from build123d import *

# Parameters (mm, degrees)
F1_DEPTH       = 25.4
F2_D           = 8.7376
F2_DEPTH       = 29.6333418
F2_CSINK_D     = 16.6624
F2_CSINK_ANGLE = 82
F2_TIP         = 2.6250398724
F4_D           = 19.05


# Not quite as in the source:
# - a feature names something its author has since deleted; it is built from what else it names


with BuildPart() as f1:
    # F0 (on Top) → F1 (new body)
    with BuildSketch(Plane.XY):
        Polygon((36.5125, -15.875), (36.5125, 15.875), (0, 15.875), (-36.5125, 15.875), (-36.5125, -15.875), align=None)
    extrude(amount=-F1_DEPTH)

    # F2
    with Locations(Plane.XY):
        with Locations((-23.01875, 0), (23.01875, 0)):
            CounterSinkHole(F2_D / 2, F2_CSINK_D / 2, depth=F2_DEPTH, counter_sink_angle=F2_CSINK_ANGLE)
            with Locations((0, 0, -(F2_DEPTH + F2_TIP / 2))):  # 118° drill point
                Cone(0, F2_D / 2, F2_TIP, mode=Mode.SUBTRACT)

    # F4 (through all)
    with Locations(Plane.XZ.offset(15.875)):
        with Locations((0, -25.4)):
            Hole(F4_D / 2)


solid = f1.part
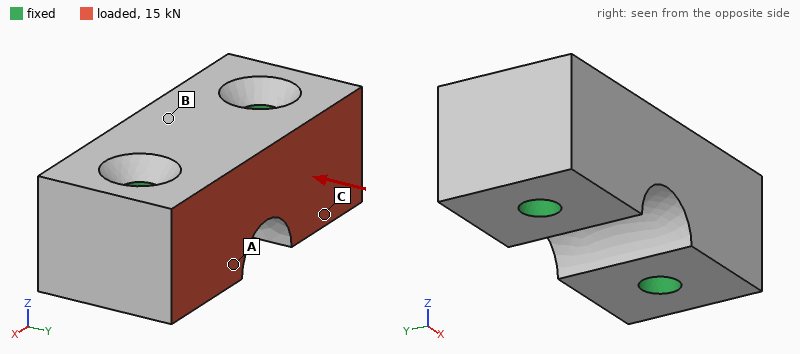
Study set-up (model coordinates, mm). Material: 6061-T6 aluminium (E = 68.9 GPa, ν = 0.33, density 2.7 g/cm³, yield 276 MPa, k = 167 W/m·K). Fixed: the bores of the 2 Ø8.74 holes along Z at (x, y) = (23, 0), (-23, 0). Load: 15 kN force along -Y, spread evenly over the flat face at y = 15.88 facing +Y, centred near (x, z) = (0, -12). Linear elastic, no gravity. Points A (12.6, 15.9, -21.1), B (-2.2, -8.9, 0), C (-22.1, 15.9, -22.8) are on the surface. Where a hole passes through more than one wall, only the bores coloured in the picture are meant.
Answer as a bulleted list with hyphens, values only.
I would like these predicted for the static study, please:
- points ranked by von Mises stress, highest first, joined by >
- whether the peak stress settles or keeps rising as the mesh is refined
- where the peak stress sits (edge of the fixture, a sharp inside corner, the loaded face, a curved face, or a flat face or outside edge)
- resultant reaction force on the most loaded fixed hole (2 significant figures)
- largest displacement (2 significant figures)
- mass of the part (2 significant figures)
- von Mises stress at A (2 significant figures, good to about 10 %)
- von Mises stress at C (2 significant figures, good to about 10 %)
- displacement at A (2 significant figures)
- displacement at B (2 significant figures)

- C > A > B
- keeps rising
- edge of the fixture
- 7.5 kN
- 6.9 µm
- 140 g
- 8.9 MPa
- 13 MPa
- 3.4 µm
- 4.4 µm
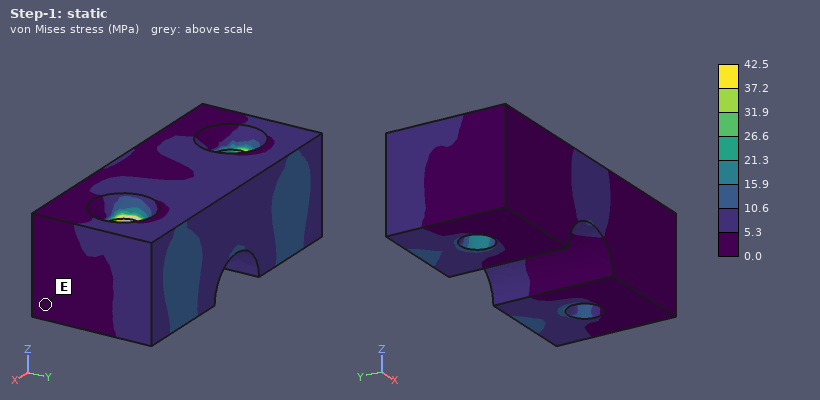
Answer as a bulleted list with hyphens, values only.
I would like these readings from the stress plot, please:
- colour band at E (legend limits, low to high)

- 0.0 to 5.3 MPa
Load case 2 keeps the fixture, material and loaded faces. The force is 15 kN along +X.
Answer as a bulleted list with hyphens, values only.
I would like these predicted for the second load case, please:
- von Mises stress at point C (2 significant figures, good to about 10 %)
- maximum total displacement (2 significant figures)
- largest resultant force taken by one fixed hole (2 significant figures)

- 16 MPa
- 14 µm
- 8.3 kN
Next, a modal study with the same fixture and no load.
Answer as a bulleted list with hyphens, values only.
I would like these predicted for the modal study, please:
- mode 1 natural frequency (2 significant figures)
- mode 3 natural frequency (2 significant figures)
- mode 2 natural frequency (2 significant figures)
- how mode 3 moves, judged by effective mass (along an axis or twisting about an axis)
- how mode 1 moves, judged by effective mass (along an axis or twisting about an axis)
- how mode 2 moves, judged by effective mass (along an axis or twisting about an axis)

- 23 kHz
- 29 kHz
- 27 kHz
- twisting about X
- along Y
- along Z
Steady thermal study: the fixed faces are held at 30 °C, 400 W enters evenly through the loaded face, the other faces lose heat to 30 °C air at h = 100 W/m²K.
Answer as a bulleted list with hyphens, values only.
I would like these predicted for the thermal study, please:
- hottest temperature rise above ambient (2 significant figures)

- 29 K
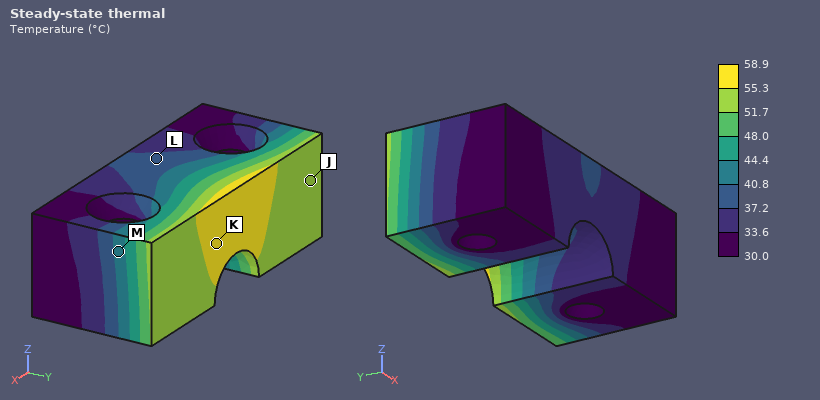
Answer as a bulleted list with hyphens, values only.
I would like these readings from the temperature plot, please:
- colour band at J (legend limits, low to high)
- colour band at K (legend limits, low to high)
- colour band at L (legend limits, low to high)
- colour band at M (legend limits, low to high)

- 51.7 to 55.3 °C
- 55.3 to 58.9 °C
- 37.2 to 40.8 °C
- 40.8 to 44.4 °C
